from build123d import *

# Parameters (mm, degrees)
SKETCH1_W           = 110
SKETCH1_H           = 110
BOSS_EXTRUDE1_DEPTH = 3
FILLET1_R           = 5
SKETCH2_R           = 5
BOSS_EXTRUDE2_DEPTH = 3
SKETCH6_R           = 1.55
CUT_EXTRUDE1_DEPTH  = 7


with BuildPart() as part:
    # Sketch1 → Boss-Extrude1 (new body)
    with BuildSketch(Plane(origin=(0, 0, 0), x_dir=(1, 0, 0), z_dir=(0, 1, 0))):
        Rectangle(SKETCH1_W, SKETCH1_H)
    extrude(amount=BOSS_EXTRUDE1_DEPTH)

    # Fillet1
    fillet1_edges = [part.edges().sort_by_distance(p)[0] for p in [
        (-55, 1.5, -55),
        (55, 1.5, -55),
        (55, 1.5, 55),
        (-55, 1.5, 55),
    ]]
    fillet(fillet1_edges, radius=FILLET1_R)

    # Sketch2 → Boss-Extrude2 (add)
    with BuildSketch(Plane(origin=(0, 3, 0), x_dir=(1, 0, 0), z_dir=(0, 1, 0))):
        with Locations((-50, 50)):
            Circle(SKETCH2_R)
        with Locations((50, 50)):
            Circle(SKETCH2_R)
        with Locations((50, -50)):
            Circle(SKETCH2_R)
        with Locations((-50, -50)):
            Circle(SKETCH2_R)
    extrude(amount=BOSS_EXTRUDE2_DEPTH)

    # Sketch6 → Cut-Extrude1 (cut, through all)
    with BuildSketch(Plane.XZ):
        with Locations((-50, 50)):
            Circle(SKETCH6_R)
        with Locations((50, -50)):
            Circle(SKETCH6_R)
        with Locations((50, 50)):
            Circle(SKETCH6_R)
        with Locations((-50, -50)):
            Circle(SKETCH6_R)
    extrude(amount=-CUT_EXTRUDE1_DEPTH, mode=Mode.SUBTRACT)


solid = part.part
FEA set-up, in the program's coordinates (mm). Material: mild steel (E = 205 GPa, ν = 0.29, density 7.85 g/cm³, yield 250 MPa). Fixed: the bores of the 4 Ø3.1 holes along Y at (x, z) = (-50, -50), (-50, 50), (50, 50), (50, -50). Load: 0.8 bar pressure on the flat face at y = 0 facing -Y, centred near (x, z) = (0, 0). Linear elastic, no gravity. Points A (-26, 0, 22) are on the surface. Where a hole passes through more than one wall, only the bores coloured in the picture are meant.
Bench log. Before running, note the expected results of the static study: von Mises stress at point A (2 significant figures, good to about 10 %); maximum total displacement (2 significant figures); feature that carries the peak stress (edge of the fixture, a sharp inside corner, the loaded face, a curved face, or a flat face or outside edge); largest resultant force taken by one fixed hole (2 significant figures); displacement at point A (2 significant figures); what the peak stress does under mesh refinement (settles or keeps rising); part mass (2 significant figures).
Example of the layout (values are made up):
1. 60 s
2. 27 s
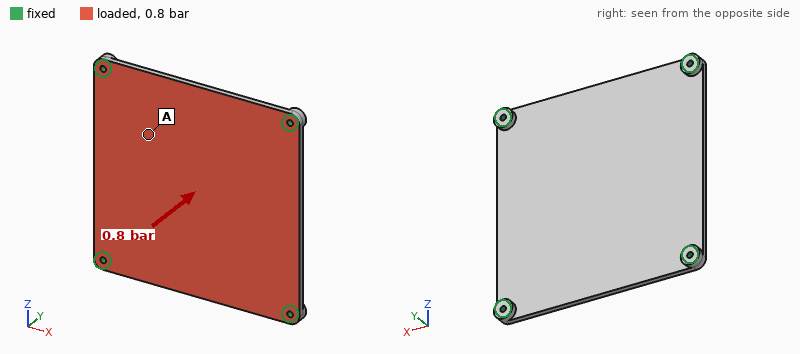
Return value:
1. 19 MPa
2. 0.12 mm
3. edge of the fixture
4. 280 N
5. 0.082 mm
6. keeps rising
7. 290 g
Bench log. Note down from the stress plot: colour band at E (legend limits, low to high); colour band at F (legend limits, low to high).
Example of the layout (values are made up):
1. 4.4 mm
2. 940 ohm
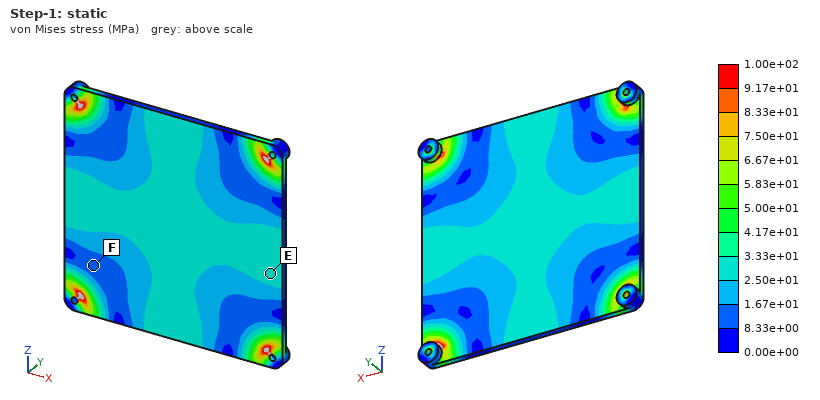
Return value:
1. 2.50e+01 to 3.33e+01 MPa
2. 8.33e+00 to 1.67e+01 MPa
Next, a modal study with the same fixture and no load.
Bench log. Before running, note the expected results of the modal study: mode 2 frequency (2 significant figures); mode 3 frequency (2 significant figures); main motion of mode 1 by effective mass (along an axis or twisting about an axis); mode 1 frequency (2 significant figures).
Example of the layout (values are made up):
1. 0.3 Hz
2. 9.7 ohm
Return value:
1. 1800 Hz
2. 1800 Hz
3. along Y
4. 1000 Hz
